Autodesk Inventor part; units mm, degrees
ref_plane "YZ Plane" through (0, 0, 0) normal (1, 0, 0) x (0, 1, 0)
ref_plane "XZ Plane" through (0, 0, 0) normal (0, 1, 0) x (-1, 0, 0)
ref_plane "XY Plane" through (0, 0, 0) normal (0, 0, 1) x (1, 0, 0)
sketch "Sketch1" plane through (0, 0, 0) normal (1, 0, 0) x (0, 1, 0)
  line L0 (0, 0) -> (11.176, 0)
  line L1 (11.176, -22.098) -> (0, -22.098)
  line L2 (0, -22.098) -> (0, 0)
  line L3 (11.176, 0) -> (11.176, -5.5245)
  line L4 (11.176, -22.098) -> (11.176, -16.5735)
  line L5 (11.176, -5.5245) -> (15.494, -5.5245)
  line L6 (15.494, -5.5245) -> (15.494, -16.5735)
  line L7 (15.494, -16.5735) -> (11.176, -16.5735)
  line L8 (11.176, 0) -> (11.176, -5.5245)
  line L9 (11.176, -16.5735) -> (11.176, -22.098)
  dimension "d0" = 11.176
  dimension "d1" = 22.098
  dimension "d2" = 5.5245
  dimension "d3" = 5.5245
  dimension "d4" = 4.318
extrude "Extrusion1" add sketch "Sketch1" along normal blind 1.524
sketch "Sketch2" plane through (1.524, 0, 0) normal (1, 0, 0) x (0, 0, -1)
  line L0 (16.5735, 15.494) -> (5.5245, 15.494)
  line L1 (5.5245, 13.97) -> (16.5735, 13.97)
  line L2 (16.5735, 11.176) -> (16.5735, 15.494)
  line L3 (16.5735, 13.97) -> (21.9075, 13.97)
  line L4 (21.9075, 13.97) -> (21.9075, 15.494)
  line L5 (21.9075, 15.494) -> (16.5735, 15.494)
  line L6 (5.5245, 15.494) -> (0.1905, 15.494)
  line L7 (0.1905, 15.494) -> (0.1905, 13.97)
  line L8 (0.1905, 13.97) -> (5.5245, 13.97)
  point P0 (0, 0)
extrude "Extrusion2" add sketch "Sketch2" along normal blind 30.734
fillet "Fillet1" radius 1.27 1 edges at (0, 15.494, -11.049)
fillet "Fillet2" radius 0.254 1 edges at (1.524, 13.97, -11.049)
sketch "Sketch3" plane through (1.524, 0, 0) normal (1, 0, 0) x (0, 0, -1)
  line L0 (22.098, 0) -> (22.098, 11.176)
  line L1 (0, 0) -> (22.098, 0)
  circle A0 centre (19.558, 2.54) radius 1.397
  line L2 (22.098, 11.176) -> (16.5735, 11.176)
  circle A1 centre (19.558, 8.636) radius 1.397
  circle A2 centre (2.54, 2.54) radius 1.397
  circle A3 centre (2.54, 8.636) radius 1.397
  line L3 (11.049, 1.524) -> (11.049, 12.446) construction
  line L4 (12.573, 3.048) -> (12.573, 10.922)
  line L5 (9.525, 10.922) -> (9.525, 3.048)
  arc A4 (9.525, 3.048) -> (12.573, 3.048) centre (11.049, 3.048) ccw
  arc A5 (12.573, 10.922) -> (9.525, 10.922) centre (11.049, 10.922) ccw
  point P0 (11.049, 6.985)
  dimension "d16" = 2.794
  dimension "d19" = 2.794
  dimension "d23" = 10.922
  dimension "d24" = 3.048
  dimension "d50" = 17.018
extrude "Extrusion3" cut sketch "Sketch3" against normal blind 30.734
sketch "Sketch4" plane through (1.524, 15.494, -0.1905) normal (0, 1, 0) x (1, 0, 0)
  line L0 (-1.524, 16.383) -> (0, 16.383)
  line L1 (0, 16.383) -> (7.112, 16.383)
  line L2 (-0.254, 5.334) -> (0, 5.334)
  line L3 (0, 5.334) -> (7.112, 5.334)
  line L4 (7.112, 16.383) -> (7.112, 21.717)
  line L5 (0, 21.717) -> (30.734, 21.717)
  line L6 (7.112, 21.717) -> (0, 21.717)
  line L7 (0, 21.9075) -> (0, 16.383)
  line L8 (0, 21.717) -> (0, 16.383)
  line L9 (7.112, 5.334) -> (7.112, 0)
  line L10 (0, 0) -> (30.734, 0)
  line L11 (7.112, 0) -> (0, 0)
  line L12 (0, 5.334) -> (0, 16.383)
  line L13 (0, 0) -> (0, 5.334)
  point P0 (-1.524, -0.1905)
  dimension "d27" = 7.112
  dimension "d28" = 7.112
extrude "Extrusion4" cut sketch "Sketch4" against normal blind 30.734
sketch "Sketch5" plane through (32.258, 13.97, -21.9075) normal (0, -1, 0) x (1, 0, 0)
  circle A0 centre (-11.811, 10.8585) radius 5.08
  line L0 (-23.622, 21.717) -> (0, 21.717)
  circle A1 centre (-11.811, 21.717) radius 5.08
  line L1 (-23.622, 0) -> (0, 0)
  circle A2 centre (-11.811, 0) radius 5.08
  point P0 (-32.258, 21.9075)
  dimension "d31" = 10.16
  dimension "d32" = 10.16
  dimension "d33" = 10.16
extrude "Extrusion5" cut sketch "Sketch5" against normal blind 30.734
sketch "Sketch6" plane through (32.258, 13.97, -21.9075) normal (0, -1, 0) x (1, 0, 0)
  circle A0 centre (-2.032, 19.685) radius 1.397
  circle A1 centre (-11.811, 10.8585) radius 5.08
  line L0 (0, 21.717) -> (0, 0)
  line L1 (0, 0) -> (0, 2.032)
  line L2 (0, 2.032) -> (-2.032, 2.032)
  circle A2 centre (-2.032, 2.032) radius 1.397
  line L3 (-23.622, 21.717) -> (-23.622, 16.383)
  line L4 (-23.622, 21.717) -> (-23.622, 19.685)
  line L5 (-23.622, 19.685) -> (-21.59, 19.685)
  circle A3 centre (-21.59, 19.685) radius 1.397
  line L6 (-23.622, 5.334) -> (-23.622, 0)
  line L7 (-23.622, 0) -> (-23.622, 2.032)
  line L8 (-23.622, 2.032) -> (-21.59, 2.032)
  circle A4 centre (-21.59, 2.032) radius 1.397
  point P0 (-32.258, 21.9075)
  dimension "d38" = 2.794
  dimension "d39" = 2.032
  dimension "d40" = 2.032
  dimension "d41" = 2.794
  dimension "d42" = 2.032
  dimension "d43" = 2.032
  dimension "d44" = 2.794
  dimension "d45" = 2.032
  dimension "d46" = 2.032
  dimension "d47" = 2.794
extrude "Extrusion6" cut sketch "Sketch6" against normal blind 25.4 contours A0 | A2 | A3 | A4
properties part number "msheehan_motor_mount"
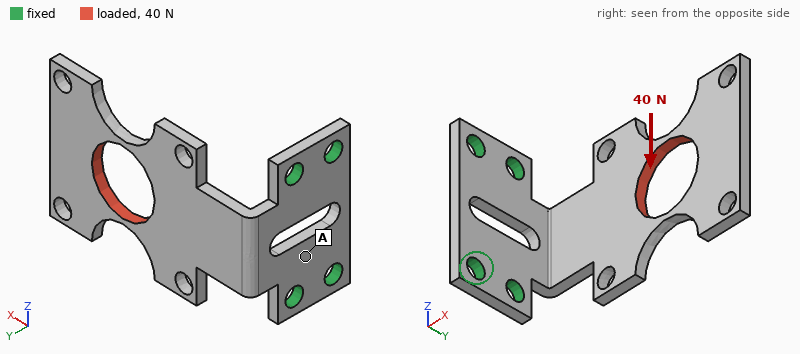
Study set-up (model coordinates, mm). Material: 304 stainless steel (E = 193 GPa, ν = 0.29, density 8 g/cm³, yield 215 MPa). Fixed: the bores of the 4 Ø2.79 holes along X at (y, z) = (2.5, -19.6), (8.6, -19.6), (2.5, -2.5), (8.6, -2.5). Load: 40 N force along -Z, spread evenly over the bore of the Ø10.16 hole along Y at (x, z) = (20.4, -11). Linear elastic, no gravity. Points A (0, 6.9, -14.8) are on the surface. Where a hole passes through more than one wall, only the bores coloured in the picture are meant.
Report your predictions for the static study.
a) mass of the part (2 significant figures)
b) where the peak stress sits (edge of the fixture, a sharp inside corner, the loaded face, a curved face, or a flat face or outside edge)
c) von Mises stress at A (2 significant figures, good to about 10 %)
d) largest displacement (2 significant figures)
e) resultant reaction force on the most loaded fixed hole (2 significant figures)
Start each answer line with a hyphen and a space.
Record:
- 7.8 g
- a curved face
- 25 MPa
- 90 µm
- 78 N
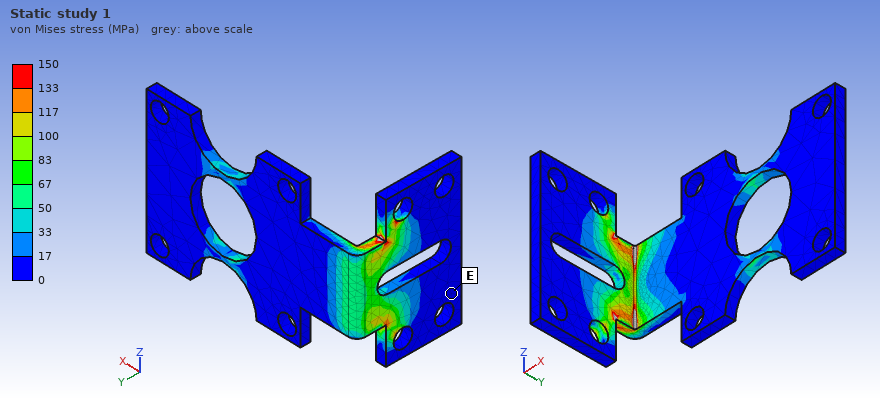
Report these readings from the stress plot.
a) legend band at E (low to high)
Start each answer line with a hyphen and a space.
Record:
- 0 to 17 MPa
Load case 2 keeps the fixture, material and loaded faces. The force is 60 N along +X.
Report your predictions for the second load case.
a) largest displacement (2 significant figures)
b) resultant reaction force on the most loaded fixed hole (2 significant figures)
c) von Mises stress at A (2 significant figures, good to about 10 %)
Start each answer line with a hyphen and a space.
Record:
- 78 µm
- 43 N
- 29 MPa
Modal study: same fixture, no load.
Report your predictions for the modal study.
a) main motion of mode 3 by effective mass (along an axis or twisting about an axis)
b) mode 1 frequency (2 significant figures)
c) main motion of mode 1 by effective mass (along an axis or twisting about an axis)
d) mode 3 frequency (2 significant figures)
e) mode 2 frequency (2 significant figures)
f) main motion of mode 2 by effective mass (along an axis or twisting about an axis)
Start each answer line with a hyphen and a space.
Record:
- twisting about X
- 730 Hz
- along Y
- 2900 Hz
- 1900 Hz
- along Z
